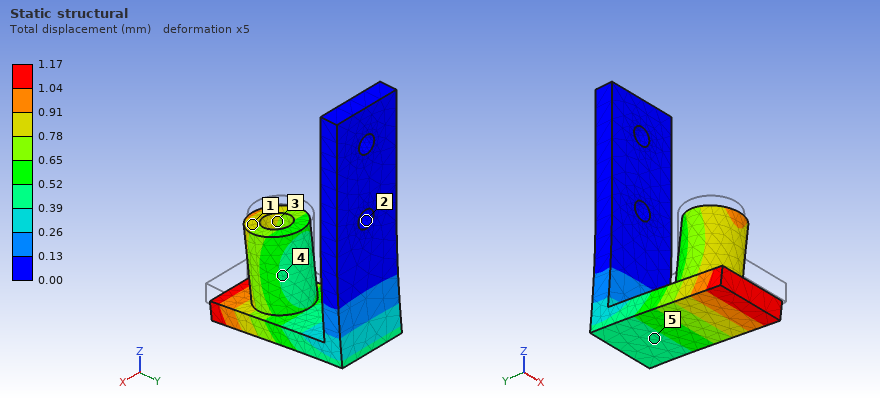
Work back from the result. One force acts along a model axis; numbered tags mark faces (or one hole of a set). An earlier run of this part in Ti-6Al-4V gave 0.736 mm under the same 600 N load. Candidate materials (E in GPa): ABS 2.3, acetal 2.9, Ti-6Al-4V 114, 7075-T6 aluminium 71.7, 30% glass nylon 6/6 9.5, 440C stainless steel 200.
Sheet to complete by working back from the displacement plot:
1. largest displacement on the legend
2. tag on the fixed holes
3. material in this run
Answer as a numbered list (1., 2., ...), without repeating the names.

1. 1.17 mm
2. 2
3. 7075-T6 aluminium
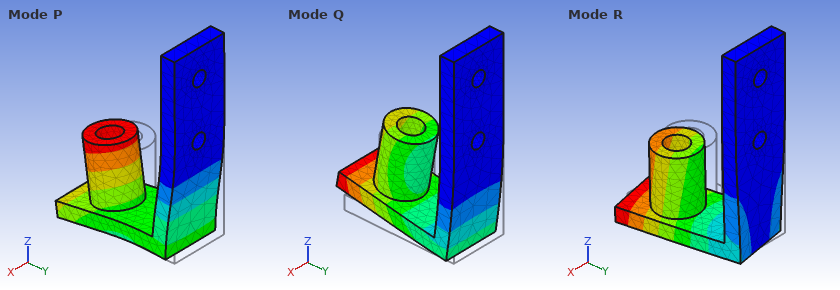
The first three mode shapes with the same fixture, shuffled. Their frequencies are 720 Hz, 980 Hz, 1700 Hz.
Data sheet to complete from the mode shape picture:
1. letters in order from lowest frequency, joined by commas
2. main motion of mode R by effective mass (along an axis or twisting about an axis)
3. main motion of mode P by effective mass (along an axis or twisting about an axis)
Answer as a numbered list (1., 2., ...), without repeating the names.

1. Q, R, P
2. along X
3. along Y
